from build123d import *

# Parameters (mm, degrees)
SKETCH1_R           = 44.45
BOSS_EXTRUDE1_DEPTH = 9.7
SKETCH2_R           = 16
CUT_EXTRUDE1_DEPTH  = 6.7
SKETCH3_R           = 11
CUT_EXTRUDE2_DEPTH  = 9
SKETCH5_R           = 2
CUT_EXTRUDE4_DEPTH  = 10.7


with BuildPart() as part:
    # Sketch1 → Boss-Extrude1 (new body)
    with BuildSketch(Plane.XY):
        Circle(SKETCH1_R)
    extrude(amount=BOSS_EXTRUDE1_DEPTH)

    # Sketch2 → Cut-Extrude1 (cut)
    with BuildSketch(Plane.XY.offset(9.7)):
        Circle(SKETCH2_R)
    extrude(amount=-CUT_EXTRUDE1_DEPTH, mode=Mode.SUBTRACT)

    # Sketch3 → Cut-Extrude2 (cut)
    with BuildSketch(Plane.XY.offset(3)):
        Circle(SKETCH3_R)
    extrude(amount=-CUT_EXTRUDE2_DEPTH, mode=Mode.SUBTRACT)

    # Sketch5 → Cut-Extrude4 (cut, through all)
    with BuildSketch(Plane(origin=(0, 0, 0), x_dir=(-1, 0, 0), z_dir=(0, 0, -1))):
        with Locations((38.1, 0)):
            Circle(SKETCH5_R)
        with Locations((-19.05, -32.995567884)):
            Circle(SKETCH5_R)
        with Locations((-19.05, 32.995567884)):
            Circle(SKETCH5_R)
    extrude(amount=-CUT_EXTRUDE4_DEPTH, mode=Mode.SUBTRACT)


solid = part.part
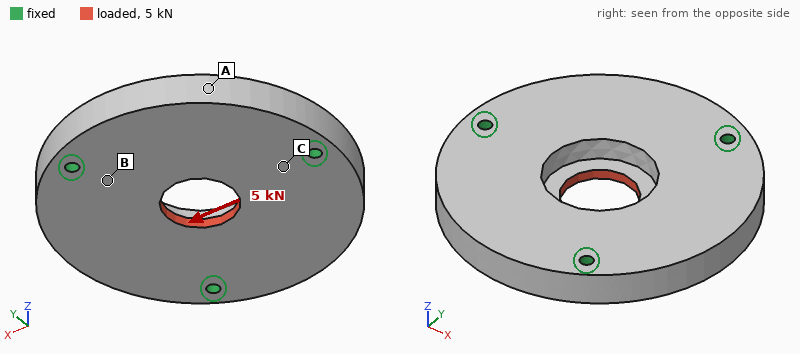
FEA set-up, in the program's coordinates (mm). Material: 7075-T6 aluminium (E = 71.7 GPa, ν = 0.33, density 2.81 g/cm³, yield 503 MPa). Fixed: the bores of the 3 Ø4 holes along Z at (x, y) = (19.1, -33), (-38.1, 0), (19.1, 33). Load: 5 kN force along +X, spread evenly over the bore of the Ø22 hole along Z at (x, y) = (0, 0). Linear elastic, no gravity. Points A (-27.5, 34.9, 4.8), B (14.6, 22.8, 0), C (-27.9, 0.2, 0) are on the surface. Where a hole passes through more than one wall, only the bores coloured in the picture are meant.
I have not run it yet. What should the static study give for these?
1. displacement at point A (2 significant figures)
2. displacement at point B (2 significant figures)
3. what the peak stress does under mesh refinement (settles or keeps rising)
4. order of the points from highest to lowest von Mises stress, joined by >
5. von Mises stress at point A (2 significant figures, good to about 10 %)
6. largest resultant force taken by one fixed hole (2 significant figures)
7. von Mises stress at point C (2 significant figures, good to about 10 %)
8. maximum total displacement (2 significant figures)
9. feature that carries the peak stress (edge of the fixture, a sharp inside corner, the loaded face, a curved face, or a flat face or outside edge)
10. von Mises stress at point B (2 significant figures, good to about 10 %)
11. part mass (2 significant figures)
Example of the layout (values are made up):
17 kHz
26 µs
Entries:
4.3 µm
3.1 µm
keeps rising
C > B > A
3.2 MPa
1.7 kN
17 MPa
11 µm
edge of the fixture
8.9 MPa
150 g
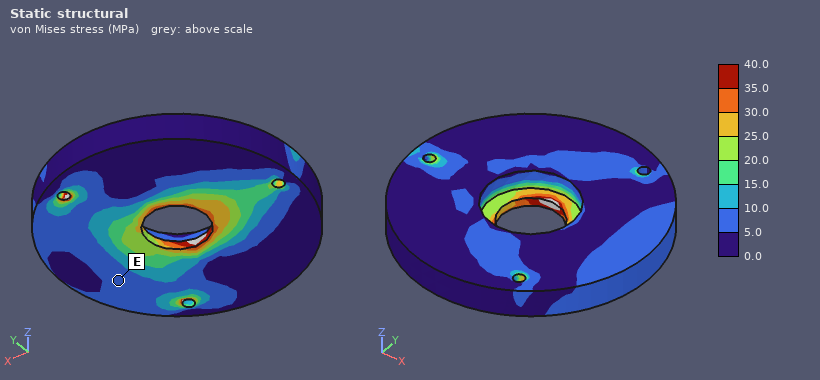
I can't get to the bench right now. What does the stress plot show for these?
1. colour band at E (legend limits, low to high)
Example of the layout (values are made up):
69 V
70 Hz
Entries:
5.0 to 10.0 MPa
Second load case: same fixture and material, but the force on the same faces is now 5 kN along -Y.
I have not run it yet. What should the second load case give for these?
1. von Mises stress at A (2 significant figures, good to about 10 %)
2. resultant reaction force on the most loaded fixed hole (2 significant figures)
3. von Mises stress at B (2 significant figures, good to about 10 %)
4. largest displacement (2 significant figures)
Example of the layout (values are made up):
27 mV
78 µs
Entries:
5.7 MPa
1.7 kN
14 MPa
10 µm
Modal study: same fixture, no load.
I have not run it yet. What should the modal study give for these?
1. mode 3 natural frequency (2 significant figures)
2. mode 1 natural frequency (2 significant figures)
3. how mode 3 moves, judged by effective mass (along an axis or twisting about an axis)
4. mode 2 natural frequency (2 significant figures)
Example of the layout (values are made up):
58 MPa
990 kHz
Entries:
7700 Hz
6600 Hz
along Z
6600 Hz
